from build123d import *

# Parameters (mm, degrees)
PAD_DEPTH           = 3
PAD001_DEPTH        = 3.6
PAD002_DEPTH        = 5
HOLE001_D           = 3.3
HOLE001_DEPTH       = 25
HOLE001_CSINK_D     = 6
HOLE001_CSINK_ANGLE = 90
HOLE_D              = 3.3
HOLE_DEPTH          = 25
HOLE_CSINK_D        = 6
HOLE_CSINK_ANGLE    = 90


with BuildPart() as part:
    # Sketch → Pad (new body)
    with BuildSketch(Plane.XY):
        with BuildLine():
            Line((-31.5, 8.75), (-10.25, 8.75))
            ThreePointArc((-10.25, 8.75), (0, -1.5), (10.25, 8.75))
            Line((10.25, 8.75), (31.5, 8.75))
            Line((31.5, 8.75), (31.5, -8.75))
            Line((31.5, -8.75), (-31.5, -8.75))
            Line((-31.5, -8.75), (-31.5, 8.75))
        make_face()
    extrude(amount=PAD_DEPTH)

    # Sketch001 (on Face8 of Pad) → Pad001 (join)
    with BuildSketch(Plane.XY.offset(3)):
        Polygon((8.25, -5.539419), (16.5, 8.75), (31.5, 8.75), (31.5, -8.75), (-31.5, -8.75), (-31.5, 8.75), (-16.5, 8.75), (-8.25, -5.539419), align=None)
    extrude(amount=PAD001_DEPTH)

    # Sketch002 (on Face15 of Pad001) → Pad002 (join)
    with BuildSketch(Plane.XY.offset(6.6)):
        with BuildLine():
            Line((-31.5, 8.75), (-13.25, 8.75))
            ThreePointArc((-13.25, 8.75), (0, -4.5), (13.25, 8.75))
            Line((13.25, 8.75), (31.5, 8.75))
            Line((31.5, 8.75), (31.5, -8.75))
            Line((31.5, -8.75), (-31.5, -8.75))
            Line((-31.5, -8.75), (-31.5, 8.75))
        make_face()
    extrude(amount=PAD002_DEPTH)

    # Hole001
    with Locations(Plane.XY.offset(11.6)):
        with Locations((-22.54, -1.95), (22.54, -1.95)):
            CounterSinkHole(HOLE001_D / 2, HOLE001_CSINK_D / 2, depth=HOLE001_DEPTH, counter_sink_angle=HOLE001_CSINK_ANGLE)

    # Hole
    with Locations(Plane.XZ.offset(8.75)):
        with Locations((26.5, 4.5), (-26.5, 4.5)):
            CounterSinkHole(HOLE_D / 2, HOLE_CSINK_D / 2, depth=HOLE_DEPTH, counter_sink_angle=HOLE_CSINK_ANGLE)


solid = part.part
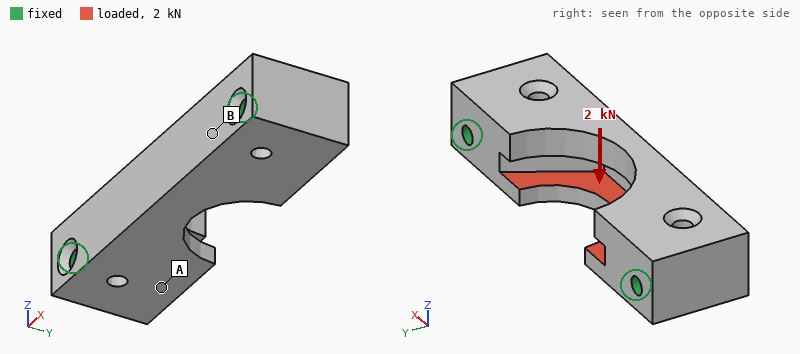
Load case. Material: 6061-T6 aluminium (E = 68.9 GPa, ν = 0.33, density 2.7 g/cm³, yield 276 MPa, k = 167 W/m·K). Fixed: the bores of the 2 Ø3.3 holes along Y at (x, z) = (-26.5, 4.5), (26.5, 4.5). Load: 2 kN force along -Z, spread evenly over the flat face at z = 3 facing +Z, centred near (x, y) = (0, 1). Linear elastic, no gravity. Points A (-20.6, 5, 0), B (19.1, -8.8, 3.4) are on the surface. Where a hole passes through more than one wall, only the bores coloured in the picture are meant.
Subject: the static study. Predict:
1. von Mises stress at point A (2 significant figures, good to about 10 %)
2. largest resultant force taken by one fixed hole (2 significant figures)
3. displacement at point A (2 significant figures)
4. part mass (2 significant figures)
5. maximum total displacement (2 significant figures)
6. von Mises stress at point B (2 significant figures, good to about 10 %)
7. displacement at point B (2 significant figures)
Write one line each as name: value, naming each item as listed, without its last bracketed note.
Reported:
von Mises stress at point A: 24 MPa
largest resultant force taken by one fixed hole: 1.0 kN
displacement at point A: 8.0 µm
part mass: 25 g
maximum total displacement: 41 µm
von Mises stress at point B: 13 MPa
displacement at point B: 7.9 µm
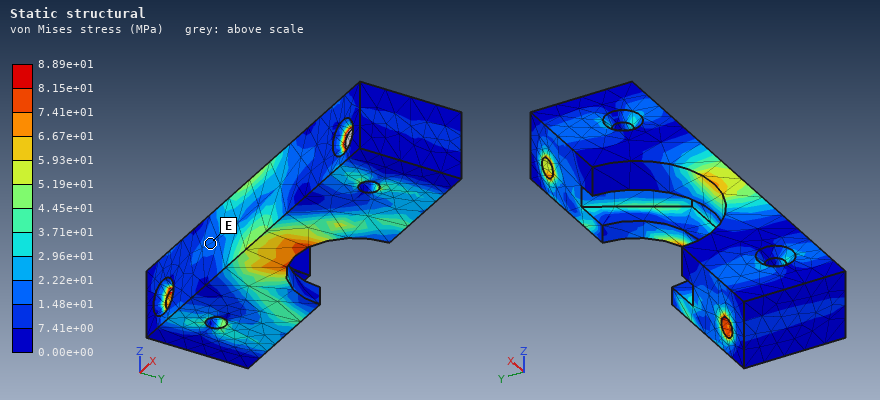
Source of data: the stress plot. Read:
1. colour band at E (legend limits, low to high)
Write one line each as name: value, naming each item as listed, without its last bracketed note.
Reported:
colour band at E: 1.48e+01 to 2.22e+01 MPa
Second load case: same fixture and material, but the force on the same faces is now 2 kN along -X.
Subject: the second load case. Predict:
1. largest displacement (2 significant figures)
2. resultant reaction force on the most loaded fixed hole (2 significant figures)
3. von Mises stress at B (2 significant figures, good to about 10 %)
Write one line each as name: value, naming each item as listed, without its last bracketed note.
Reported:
largest displacement: 4.4 µm
resultant reaction force on the most loaded fixed hole: 1.0 kN
von Mises stress at B: 7.1 MPa
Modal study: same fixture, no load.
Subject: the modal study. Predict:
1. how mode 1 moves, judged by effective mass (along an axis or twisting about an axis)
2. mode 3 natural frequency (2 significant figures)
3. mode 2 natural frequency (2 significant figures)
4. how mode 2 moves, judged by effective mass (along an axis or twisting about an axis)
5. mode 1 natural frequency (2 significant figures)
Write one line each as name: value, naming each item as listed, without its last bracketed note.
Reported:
how mode 1 moves, judged by effective mass: along Z
mode 3 natural frequency: 27 kHz
mode 2 natural frequency: 24 kHz
how mode 2 moves, judged by effective mass: along Y
mode 1 natural frequency: 15 kHz
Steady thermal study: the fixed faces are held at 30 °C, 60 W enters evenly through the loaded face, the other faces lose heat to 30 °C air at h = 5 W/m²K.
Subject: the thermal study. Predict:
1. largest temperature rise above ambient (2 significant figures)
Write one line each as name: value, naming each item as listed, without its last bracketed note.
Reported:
largest temperature rise above ambient: 33 K
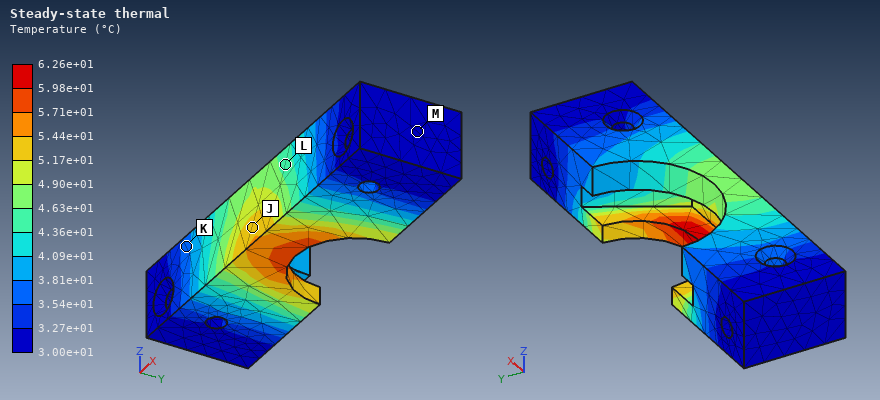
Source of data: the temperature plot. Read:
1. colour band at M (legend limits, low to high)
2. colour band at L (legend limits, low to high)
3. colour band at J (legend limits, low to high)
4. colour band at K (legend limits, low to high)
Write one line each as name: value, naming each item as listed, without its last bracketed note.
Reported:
colour band at M: 3.00e+01 to 3.27e+01 °C
colour band at L: 4.36e+01 to 4.63e+01 °C
colour band at J: 5.17e+01 to 5.44e+01 °C
colour band at K: 3.54e+01 to 3.81e+01 °C
